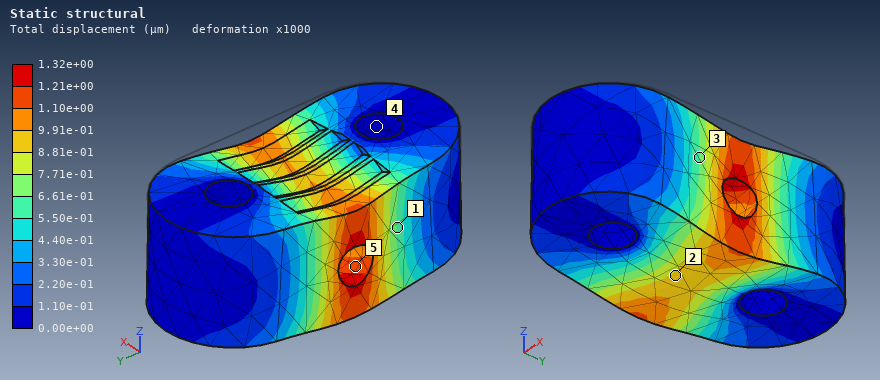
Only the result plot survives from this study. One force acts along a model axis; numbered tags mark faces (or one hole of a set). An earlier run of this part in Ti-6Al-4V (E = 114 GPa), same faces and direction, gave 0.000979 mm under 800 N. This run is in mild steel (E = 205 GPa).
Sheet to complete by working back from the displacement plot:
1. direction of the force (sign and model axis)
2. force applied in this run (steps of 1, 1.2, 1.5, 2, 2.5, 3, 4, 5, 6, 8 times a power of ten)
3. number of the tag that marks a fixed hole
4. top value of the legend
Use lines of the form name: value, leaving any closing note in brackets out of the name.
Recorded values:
direction of the force: -Z
force applied in this run: 2 kN
number of the tag that marks a fixed hole: 4
top value of the legend: 1.32e+00 µm
